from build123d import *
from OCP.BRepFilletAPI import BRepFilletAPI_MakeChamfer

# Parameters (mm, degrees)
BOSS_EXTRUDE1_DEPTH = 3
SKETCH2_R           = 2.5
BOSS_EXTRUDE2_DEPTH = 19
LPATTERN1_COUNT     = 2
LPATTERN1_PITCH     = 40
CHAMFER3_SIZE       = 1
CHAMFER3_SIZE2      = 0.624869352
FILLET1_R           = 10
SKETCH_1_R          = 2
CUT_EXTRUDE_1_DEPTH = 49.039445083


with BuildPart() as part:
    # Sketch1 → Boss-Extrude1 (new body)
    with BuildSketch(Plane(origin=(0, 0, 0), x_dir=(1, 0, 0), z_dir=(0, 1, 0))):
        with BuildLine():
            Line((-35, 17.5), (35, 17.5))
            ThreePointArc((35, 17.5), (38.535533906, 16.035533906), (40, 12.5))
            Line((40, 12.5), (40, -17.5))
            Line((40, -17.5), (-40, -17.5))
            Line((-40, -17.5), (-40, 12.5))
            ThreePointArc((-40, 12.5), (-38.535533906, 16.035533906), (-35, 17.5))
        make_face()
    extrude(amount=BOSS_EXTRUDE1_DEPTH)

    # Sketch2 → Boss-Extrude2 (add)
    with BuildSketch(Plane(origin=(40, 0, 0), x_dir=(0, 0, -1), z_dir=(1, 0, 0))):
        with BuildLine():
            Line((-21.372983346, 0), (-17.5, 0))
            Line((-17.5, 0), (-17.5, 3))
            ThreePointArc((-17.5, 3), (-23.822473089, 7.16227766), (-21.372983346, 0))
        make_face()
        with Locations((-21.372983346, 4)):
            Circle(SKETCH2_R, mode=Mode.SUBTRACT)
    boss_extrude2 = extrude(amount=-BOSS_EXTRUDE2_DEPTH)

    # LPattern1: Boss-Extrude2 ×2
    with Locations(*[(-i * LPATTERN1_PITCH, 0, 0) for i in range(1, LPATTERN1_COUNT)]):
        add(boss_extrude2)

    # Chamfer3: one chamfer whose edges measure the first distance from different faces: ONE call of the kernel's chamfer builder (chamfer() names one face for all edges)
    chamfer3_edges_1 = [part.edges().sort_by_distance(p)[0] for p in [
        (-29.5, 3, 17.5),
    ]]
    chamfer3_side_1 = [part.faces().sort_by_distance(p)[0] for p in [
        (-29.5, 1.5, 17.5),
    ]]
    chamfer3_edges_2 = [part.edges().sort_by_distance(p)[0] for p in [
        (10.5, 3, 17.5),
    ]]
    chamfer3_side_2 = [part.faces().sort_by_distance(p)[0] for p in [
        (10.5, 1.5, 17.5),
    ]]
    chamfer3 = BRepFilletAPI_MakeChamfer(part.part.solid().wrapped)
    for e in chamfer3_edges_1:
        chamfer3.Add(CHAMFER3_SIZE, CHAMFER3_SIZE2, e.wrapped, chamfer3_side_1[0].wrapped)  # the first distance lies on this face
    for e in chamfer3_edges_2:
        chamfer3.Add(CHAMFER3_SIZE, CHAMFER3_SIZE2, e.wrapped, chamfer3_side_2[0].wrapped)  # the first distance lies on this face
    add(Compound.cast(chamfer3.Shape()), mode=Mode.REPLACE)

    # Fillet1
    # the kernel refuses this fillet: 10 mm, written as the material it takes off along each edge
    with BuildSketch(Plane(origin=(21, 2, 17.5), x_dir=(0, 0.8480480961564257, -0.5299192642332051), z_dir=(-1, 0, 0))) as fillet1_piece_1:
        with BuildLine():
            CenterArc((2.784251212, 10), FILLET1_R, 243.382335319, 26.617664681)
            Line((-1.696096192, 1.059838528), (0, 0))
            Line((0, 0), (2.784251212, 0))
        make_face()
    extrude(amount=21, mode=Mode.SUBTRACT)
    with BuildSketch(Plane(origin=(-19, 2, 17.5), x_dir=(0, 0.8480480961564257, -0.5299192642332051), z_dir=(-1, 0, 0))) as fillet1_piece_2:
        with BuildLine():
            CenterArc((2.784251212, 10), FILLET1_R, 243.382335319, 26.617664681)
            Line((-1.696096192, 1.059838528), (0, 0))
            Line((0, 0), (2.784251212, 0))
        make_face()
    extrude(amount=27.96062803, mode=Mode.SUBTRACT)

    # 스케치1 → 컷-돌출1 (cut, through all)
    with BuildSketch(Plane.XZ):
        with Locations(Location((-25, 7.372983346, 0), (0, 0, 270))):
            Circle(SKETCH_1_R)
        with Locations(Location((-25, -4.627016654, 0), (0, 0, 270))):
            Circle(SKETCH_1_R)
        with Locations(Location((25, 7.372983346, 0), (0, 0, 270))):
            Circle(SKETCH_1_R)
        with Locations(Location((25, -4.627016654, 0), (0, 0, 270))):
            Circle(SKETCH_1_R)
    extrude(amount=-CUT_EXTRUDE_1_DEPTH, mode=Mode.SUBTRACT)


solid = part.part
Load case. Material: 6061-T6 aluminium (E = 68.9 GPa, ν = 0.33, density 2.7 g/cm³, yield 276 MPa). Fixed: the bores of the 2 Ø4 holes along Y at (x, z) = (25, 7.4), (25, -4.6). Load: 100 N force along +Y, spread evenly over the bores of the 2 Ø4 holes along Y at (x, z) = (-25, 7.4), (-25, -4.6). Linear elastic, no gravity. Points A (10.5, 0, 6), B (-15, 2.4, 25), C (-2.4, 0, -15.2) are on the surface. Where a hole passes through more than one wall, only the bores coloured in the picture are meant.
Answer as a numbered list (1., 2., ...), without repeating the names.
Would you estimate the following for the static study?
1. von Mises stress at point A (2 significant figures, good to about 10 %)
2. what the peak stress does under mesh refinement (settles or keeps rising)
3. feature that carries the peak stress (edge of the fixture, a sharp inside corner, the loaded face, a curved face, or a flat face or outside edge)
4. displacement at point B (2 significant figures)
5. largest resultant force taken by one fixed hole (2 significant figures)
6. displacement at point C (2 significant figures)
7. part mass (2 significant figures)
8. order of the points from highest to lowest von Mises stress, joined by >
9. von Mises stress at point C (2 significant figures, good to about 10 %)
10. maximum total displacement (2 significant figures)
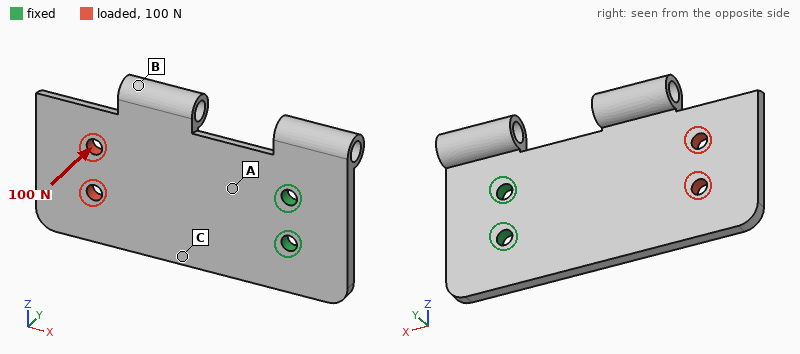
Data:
1. 63 MPa
2. keeps rising
3. edge of the fixture
4. 0.50 mm
5. 52 N
6. 0.25 mm
7. 26 g
8. A > C > B
9. 42 MPa
10. 1.0 mm
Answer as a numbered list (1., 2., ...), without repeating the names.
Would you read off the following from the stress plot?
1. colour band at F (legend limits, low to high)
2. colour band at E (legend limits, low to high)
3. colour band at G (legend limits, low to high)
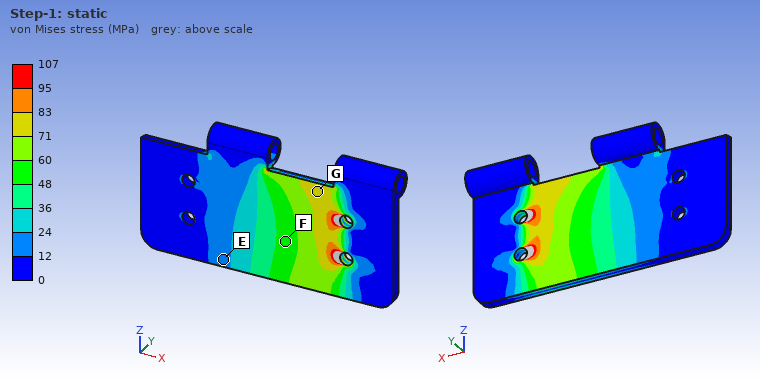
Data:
1. 48 to 60 MPa
2. 12 to 24 MPa
3. 71 to 83 MPa
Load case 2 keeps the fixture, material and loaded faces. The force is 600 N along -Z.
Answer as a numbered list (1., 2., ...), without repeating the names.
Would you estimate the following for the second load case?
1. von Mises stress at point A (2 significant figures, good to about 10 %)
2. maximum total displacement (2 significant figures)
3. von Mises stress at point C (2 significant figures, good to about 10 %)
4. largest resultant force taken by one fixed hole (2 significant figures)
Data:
1. 22 MPa
2. 0.10 mm
3. 19 MPa
4. 2.0 kN
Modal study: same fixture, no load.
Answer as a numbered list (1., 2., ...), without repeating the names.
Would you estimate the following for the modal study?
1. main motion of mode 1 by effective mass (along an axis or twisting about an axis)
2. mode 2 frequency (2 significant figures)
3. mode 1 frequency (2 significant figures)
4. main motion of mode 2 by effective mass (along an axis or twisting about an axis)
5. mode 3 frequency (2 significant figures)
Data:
1. along Y
2. 1900 Hz
3. 590 Hz
4. twisting about X
5. 3600 Hz
